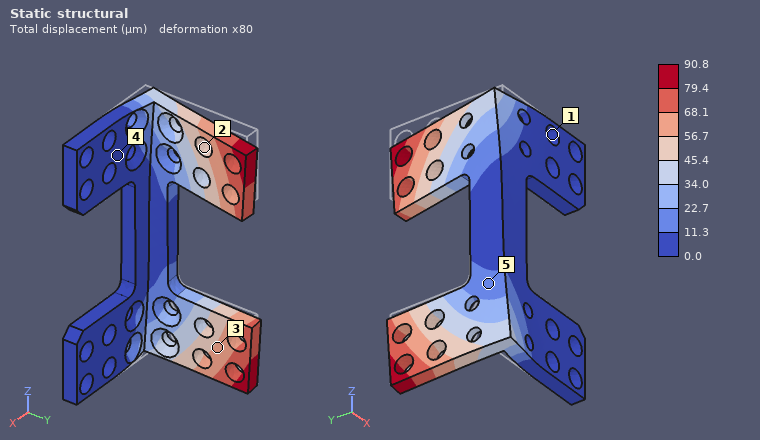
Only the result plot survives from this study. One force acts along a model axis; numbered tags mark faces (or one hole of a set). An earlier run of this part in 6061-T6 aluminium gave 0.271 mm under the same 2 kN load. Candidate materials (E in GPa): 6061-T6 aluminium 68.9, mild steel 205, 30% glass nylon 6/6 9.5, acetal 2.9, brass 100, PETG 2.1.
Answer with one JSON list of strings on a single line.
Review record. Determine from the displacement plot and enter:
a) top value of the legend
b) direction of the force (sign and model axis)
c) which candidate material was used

["90.8 µm", "-Z", "mild steel"]
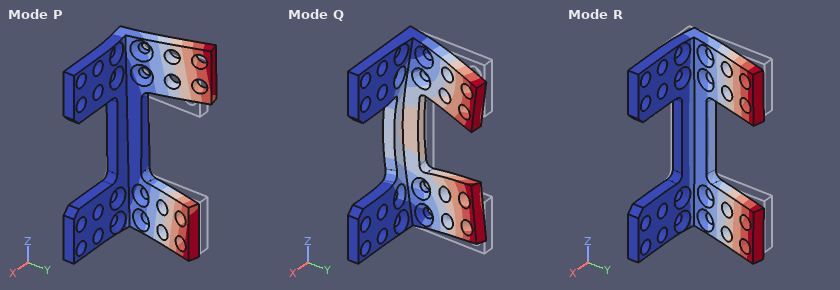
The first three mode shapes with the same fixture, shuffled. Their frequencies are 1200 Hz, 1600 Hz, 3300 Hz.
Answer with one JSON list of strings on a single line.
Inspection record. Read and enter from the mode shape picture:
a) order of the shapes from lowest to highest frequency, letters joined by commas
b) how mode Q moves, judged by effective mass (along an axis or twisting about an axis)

["R, P, Q", "along Y"]
